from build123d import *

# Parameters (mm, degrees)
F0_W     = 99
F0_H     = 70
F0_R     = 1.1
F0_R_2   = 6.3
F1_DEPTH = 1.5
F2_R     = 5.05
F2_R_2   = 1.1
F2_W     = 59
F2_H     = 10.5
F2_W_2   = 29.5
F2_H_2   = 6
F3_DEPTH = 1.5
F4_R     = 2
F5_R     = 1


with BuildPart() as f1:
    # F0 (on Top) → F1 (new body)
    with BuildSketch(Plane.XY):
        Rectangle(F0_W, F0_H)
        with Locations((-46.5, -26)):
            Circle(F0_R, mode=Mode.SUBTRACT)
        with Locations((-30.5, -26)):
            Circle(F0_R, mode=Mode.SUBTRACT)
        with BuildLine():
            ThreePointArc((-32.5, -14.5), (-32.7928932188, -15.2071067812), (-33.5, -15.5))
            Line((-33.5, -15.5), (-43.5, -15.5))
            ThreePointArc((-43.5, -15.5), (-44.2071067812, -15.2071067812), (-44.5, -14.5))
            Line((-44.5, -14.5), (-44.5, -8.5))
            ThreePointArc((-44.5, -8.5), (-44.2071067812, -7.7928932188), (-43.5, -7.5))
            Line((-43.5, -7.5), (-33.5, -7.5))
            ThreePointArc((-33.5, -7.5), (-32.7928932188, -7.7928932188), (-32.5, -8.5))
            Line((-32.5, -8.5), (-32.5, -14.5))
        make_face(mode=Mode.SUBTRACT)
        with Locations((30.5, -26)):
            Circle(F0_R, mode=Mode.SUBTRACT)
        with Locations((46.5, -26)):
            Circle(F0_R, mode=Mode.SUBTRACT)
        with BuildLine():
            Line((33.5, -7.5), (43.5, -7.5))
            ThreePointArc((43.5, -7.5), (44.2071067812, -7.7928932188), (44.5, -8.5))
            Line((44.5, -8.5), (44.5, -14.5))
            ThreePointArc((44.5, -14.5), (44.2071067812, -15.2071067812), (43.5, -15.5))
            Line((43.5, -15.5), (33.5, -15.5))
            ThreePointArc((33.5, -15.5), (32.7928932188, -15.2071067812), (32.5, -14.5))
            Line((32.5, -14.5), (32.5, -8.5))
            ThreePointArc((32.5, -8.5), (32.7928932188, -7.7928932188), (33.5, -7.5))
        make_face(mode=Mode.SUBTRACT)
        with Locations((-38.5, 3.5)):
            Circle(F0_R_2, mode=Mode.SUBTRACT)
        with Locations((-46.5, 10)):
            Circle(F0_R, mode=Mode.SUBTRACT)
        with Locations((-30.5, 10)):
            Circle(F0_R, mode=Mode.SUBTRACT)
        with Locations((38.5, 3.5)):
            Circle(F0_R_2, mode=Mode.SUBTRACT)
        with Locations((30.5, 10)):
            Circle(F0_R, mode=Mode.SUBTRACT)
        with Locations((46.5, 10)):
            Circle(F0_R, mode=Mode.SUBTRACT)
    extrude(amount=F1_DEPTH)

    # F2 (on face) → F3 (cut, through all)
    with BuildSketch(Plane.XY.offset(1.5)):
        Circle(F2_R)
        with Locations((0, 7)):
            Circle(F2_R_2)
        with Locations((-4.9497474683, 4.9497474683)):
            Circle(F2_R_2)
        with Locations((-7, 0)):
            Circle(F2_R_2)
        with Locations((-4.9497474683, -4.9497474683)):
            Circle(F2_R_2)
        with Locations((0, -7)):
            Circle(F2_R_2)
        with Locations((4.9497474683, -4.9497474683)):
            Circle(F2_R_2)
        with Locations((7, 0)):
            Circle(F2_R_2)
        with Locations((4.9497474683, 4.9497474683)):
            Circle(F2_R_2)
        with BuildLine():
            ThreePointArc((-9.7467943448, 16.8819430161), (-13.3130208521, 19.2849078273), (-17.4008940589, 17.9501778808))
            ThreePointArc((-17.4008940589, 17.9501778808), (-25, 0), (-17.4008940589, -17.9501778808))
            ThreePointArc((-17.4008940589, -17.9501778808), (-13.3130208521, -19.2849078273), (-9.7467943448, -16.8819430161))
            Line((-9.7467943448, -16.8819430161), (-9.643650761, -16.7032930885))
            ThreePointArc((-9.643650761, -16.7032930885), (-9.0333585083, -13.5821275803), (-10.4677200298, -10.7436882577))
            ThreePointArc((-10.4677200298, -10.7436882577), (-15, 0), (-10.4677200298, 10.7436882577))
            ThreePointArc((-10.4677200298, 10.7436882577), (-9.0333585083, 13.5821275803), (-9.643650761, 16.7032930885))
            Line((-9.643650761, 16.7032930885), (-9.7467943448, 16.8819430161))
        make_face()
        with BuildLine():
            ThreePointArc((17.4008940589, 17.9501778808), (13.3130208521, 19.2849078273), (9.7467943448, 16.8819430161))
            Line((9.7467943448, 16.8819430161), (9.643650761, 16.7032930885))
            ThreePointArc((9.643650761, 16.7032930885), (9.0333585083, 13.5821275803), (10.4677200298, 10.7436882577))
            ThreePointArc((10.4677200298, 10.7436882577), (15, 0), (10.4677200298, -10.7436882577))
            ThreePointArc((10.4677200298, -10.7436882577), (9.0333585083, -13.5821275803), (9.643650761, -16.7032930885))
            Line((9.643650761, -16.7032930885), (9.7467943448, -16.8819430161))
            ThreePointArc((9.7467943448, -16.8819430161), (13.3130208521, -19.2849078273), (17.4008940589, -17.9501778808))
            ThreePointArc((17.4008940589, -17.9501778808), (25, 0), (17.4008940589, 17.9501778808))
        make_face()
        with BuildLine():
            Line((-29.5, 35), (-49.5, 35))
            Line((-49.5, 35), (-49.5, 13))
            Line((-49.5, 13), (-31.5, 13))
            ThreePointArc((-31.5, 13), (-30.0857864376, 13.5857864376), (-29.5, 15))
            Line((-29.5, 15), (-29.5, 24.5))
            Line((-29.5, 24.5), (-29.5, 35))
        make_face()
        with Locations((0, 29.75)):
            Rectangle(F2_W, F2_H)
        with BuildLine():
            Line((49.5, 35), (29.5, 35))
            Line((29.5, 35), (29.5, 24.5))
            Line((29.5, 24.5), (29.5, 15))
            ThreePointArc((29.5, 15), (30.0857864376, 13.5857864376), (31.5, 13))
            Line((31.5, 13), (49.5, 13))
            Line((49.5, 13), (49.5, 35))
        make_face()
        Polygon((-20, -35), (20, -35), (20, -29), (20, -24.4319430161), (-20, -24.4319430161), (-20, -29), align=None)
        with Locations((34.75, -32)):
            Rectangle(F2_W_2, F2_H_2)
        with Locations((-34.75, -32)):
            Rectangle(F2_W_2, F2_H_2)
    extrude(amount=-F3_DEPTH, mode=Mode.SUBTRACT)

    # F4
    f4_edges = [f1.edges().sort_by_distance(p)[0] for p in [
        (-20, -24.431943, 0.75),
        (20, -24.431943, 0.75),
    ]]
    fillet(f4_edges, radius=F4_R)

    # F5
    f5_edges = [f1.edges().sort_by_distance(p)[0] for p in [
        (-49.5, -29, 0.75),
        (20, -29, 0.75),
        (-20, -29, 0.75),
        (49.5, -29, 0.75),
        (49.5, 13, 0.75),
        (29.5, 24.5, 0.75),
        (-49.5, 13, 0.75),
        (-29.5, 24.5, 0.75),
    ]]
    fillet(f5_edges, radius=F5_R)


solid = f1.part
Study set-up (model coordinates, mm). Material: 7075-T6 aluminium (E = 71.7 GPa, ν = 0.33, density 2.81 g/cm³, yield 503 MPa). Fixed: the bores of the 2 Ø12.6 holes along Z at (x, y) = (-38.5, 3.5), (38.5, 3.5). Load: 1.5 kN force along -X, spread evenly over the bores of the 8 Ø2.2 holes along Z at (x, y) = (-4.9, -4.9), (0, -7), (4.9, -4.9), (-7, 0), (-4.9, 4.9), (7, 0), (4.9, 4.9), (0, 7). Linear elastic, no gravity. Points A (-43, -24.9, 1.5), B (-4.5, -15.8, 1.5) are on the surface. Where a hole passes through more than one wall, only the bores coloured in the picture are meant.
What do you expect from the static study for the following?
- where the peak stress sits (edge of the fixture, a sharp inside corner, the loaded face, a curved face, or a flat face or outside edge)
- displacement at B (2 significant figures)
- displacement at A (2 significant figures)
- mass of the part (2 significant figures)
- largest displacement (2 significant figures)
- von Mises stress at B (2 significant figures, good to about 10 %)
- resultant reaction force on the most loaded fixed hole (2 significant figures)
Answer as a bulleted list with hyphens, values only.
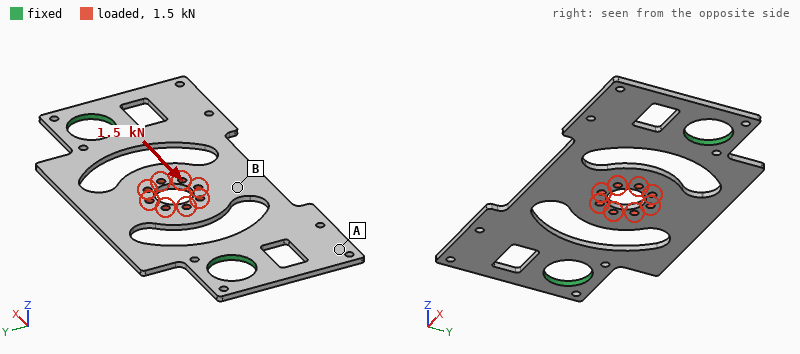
- a curved face
- 66 µm
- 43 µm
- 14 g
- 89 µm
- 61 MPa
- 750 N
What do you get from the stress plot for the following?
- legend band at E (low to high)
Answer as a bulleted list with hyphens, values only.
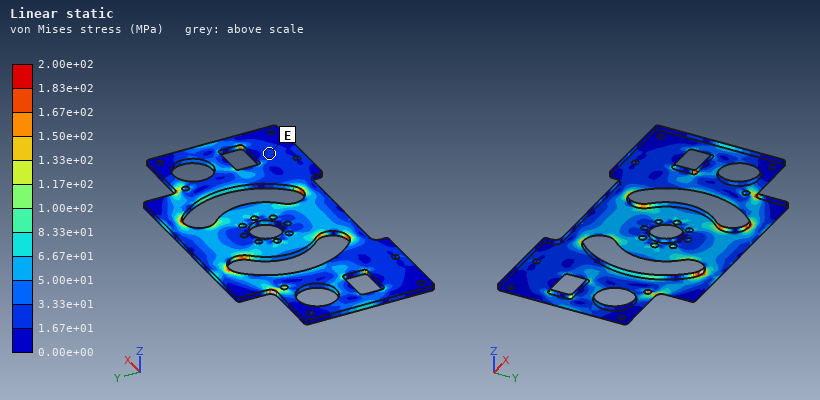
- 1.67e+01 to 3.33e+01 MPa
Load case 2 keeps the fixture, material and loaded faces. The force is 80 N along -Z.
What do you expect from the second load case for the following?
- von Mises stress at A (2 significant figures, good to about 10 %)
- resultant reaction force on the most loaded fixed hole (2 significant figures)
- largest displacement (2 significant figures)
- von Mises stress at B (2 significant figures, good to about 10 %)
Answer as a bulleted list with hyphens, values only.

- 12 MPa
- 40 N
- 0.52 mm
- 40 MPa
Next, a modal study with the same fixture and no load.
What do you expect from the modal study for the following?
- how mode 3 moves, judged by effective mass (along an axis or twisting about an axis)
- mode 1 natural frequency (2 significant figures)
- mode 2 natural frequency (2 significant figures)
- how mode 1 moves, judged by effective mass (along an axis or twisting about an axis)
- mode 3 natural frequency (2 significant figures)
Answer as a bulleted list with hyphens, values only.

- twisting about Y
- 890 Hz
- 1100 Hz
- along Z
- 1400 Hz
